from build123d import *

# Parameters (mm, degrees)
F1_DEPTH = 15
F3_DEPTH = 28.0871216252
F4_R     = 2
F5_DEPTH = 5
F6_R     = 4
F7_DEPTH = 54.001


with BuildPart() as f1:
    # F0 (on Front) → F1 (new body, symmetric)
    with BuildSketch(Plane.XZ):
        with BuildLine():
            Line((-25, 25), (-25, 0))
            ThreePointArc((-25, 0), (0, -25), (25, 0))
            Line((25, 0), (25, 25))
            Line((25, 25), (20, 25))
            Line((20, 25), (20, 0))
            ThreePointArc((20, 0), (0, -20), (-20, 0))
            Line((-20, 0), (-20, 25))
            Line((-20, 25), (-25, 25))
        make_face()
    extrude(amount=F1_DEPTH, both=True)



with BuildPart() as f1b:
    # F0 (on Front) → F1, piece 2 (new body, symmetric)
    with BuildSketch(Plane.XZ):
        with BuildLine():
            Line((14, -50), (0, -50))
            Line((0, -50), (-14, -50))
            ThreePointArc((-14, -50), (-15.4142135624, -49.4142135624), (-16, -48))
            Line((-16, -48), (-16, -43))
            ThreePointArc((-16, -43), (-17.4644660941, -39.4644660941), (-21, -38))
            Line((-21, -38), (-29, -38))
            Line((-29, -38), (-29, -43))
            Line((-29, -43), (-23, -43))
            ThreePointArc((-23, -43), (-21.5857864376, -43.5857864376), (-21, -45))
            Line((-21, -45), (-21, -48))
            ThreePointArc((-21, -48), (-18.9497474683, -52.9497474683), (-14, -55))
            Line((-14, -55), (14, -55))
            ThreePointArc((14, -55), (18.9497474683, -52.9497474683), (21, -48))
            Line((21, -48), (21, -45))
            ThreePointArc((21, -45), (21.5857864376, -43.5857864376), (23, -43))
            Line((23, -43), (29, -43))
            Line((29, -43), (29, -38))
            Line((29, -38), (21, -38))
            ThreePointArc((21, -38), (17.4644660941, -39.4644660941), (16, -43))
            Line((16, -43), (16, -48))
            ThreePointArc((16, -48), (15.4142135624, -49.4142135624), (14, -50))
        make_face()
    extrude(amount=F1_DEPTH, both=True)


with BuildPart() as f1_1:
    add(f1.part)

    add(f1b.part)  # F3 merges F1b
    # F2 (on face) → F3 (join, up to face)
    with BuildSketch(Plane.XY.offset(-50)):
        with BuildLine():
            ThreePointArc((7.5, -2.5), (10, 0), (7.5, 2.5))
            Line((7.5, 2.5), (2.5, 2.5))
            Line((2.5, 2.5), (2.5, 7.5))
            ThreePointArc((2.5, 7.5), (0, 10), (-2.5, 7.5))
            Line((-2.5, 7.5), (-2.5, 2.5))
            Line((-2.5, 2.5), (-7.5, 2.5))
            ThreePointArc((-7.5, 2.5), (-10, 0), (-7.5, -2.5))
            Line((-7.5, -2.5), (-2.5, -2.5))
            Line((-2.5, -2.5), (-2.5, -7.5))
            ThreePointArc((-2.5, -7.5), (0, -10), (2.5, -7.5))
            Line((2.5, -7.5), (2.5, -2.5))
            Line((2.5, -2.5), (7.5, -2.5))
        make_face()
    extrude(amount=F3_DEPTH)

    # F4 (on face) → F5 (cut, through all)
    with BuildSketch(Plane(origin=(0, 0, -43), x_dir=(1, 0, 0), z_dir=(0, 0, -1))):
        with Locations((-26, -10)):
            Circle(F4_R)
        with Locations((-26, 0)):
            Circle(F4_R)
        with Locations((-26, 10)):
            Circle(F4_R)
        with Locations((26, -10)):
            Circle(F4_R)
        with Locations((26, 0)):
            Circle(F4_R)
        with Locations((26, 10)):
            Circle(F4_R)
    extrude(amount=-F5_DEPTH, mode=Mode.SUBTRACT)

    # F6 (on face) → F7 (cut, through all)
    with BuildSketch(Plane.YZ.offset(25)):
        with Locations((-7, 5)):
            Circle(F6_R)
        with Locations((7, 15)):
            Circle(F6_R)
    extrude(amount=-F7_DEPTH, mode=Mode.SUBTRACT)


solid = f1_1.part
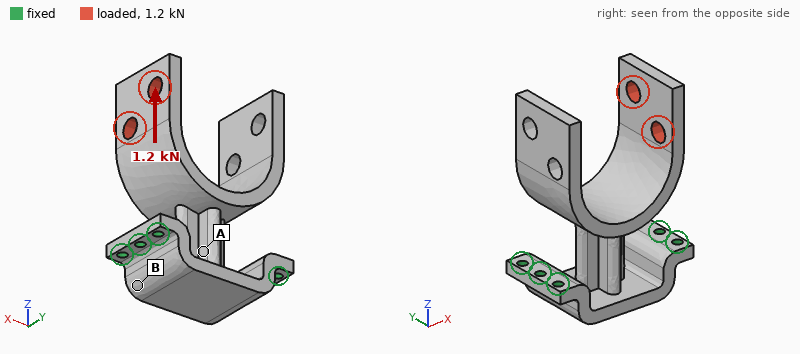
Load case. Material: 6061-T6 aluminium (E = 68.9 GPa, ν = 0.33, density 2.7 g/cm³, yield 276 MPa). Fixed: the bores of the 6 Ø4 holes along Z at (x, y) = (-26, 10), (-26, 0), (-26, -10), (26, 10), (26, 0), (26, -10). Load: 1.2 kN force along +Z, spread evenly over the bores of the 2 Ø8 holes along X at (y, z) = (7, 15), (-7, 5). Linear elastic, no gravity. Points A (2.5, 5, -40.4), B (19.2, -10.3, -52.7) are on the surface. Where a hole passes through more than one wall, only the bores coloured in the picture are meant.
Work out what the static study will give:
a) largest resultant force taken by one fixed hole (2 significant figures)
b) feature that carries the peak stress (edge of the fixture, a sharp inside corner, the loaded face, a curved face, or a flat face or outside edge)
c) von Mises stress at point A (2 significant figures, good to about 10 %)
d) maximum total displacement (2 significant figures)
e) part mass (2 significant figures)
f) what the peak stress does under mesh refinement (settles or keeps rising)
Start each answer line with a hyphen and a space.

- 520 N
- a sharp inside corner
- 29 MPa
- 0.92 mm
- 87 g
- keeps rising
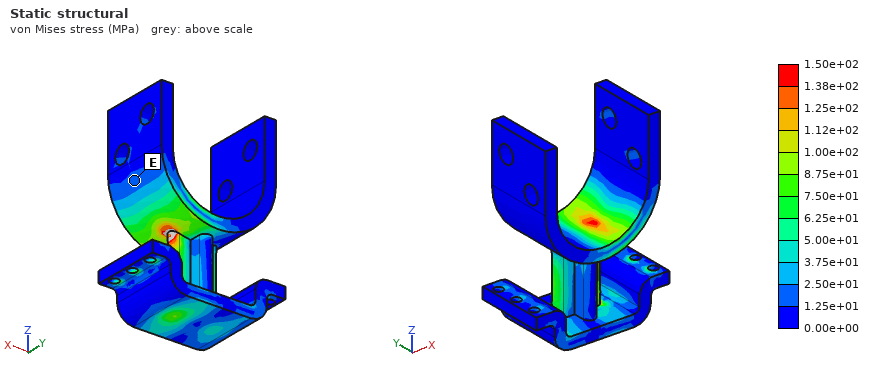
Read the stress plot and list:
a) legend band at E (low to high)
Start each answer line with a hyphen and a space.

- 1.25e+01 to 2.50e+01 MPa
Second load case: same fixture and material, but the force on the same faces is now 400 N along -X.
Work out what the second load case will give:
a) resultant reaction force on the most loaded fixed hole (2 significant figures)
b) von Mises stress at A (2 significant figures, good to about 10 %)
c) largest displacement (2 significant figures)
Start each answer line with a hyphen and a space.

- 260 N
- 17 MPa
- 0.92 mm
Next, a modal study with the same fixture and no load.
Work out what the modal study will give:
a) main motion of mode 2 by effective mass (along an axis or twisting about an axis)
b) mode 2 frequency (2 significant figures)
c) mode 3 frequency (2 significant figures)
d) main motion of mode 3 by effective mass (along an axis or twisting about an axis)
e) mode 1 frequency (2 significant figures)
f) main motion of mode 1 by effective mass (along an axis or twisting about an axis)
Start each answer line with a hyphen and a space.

- along Y
- 940 Hz
- 1400 Hz
- twisting about Z
- 890 Hz
- along X
